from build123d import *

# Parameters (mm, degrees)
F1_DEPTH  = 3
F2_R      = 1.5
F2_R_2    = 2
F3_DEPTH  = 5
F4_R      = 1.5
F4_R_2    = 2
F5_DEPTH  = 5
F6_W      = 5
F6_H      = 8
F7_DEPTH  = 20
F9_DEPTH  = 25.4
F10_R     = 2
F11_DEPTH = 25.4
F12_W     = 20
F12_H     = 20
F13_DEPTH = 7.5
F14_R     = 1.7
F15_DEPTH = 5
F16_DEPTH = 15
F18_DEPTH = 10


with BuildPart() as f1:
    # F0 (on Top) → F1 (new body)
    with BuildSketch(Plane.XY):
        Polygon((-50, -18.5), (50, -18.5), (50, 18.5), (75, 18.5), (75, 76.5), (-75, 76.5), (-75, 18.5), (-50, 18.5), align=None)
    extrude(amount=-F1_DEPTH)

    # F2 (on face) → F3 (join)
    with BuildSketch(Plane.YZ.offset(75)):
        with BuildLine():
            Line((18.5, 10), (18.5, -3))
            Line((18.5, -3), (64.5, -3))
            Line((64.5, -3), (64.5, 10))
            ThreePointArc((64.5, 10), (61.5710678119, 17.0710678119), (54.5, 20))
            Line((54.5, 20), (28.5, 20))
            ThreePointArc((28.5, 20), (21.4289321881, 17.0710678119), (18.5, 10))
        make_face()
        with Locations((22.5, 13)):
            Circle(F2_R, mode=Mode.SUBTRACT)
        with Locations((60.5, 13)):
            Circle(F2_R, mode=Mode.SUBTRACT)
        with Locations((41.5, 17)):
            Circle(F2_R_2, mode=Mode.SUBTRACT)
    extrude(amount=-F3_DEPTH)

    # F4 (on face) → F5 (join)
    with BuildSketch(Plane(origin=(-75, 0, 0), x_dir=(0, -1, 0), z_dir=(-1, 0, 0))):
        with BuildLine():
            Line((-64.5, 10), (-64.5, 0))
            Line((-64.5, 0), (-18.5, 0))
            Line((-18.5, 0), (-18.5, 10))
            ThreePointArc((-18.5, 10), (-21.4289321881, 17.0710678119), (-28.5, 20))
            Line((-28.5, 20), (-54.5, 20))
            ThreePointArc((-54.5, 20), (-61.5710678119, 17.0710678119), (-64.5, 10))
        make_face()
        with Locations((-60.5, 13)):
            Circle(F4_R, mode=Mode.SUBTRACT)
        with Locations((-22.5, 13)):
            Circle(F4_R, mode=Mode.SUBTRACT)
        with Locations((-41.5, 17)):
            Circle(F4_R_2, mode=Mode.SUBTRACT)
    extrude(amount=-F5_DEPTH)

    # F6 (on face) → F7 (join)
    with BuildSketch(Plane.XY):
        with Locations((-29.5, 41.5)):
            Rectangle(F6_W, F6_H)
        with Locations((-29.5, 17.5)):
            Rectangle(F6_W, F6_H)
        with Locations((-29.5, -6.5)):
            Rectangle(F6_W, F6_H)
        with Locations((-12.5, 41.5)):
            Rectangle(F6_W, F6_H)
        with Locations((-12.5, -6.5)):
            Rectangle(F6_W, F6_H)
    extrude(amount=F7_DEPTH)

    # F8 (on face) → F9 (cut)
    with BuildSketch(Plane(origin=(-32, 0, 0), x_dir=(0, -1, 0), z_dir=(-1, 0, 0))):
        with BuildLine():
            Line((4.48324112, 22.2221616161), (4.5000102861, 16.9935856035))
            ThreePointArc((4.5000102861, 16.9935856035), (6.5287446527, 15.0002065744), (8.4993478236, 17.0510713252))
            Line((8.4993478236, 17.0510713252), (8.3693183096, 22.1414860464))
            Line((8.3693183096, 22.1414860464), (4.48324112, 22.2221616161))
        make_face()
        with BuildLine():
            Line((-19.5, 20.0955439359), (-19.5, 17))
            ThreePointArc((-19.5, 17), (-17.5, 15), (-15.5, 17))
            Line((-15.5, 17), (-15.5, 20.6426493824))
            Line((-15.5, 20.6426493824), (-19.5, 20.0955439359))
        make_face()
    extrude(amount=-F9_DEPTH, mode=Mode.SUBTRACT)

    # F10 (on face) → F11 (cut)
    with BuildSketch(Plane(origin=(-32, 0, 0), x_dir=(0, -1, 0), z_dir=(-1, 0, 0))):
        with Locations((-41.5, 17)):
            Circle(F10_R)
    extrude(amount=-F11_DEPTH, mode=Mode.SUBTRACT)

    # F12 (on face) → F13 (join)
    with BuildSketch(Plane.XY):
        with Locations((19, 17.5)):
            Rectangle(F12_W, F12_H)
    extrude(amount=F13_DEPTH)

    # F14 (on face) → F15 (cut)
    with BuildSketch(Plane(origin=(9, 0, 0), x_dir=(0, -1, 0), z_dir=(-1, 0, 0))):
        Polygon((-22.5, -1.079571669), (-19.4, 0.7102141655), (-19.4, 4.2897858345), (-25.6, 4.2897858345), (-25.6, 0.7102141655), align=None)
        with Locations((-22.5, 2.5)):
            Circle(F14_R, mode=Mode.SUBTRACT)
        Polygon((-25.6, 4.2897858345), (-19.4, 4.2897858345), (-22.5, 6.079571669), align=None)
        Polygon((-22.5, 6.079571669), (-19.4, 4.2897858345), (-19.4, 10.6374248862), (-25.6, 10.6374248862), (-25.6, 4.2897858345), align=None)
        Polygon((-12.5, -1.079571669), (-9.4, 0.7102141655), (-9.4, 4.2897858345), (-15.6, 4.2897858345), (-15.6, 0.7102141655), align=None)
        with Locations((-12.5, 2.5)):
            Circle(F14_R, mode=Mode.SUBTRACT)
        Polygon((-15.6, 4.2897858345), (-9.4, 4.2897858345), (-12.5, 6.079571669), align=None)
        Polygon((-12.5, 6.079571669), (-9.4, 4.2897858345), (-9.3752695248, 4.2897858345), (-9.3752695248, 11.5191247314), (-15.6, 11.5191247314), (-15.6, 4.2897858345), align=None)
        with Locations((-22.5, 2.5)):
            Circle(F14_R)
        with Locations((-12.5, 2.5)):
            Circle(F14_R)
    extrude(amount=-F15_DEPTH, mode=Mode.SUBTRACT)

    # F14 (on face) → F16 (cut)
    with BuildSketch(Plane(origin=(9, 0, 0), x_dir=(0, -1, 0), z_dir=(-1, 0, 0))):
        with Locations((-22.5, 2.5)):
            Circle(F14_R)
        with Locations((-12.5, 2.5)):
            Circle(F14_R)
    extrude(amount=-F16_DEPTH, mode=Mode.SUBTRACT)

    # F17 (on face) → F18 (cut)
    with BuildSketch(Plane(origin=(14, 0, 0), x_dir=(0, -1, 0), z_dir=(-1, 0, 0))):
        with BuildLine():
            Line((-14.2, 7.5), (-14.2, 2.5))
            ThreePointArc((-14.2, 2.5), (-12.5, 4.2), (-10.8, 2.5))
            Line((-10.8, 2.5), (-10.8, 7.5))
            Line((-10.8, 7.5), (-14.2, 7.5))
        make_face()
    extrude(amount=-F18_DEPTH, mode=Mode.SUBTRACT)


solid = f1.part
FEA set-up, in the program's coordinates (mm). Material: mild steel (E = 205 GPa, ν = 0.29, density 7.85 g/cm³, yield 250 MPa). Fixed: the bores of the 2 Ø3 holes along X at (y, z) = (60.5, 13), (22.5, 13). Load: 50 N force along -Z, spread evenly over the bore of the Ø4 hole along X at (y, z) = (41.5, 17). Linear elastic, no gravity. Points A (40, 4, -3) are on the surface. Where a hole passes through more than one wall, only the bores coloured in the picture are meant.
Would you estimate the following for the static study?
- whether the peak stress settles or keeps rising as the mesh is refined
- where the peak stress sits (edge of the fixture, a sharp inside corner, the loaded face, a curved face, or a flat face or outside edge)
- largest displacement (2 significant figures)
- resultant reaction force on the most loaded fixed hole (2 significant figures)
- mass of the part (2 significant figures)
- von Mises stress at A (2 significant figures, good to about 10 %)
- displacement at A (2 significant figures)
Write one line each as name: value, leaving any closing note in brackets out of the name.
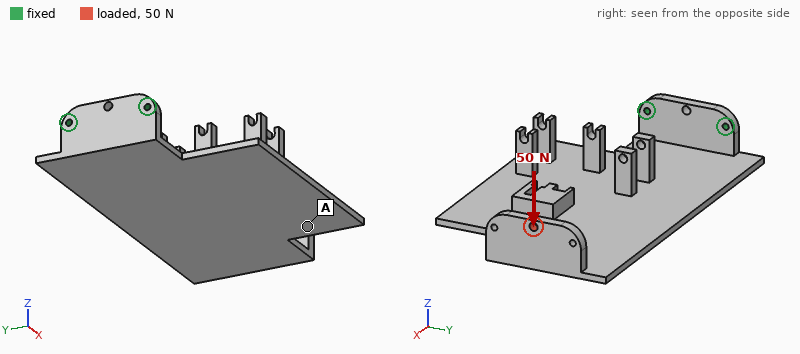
whether the peak stress settles or keeps rising as the mesh is refined: keeps rising
where the peak stress sits: edge of the fixture
largest displacement: 1.8 mm
resultant reaction force on the most loaded fixed hole: 66 N
mass of the part: 400 g
von Mises stress at A: 12 MPa
displacement at A: 1.2 mm
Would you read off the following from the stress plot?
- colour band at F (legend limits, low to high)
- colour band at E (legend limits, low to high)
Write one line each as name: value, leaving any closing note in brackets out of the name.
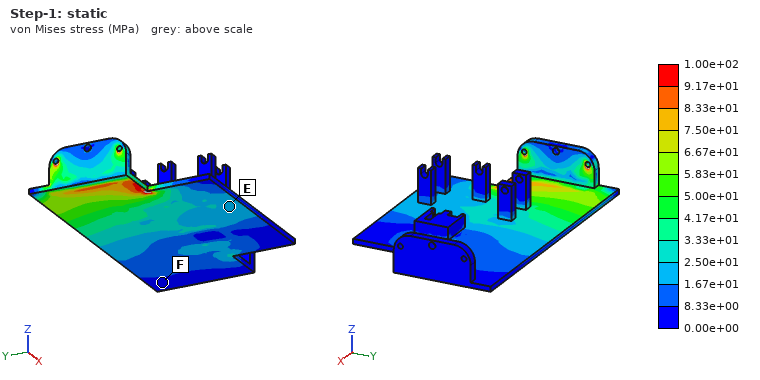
colour band at F: 0.00e+00 to 8.33e+00 MPa
colour band at E: 1.67e+01 to 2.50e+01 MPa
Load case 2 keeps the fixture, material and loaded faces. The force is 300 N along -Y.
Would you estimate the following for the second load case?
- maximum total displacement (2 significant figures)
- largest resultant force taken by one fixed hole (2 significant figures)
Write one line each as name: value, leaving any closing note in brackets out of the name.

maximum total displacement: 0.69 mm
largest resultant force taken by one fixed hole: 1.2 kN
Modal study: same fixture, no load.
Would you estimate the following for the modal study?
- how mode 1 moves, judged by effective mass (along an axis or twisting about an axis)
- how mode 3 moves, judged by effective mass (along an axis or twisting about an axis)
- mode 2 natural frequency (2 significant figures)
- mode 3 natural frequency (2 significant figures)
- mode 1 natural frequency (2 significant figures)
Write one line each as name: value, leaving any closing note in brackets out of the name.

how mode 1 moves, judged by effective mass: along Z
how mode 3 moves, judged by effective mass: along Y
mode 2 natural frequency: 290 Hz
mode 3 natural frequency: 470 Hz
mode 1 natural frequency: 81 Hz
